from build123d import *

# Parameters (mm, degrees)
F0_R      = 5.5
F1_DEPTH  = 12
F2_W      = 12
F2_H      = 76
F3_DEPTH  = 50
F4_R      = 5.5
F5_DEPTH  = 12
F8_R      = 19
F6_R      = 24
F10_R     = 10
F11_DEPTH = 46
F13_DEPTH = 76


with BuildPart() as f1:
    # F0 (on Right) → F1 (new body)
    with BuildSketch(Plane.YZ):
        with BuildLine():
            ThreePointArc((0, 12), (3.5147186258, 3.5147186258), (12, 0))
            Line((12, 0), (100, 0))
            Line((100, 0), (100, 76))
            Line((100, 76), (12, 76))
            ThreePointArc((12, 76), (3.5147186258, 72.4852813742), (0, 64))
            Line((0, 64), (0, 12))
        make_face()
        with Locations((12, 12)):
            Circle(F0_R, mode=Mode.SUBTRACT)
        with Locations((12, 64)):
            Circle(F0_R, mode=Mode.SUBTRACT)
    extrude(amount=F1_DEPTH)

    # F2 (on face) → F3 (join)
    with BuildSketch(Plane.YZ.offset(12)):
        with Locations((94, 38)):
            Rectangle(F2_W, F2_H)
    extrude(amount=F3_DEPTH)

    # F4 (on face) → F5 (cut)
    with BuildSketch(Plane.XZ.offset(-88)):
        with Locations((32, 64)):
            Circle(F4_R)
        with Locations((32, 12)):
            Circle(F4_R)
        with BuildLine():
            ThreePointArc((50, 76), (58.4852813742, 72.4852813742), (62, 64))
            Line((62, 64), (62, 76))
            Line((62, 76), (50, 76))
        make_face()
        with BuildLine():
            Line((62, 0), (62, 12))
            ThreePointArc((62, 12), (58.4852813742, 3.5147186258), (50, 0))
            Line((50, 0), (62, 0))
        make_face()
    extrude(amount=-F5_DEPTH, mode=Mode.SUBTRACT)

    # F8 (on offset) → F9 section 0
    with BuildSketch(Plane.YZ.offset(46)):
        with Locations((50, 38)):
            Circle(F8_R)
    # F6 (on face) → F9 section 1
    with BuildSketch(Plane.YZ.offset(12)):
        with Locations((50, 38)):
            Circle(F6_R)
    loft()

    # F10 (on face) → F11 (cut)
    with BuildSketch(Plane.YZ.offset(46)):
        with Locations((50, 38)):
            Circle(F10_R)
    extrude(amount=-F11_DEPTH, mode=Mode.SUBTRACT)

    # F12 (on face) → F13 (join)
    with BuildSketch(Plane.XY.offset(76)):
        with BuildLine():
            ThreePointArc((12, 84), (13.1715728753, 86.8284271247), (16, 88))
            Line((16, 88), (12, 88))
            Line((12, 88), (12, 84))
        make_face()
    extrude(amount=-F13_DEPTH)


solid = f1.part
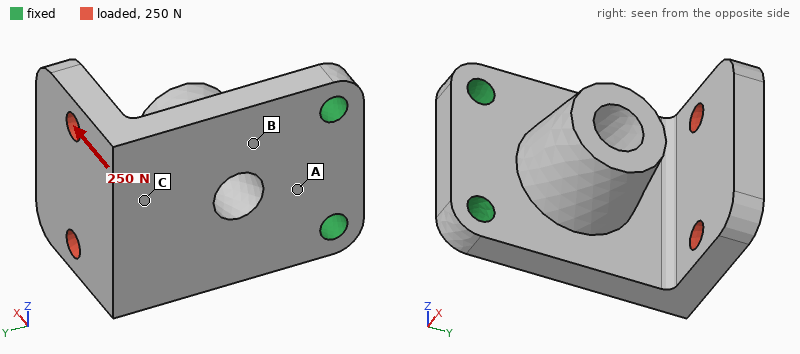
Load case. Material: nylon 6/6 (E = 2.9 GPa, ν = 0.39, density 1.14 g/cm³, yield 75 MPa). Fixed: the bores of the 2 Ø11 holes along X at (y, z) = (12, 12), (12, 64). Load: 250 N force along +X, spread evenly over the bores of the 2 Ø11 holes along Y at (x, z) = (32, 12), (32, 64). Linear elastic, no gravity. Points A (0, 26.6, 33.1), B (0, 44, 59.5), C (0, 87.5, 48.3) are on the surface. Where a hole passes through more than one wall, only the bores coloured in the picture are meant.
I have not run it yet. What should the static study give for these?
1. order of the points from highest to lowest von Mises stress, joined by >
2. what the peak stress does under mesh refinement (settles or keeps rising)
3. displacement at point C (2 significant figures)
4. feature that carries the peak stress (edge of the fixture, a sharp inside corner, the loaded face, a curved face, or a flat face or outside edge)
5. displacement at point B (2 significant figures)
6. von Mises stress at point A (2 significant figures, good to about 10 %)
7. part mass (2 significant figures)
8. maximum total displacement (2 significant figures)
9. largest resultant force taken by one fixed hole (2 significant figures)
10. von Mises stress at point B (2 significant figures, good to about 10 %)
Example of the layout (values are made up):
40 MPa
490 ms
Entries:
A > B > C
keeps rising
0.92 mm
edge of the fixture
0.27 mm
6.6 MPa
190 g
1.5 mm
130 N
3.3 MPa
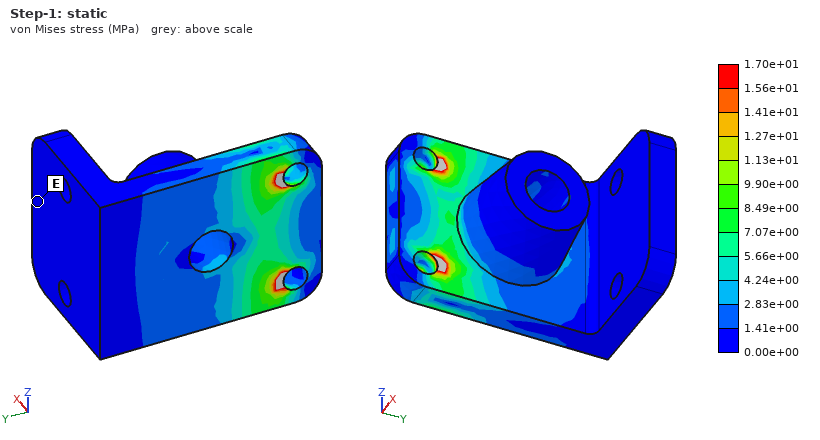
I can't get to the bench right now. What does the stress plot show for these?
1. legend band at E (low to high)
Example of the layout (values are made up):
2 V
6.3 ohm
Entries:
0.00e+00 to 1.41e+00 MPa
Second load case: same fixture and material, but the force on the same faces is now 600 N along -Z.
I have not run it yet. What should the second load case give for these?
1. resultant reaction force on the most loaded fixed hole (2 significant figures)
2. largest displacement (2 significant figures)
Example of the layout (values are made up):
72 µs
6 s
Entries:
960 N
0.73 mm
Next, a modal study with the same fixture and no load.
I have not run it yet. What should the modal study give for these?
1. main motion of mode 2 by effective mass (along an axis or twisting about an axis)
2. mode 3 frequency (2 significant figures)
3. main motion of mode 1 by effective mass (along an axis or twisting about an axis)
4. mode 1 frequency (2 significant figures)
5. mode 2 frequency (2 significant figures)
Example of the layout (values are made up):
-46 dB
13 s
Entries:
along Z
750 Hz
along X
240 Hz
600 Hz
